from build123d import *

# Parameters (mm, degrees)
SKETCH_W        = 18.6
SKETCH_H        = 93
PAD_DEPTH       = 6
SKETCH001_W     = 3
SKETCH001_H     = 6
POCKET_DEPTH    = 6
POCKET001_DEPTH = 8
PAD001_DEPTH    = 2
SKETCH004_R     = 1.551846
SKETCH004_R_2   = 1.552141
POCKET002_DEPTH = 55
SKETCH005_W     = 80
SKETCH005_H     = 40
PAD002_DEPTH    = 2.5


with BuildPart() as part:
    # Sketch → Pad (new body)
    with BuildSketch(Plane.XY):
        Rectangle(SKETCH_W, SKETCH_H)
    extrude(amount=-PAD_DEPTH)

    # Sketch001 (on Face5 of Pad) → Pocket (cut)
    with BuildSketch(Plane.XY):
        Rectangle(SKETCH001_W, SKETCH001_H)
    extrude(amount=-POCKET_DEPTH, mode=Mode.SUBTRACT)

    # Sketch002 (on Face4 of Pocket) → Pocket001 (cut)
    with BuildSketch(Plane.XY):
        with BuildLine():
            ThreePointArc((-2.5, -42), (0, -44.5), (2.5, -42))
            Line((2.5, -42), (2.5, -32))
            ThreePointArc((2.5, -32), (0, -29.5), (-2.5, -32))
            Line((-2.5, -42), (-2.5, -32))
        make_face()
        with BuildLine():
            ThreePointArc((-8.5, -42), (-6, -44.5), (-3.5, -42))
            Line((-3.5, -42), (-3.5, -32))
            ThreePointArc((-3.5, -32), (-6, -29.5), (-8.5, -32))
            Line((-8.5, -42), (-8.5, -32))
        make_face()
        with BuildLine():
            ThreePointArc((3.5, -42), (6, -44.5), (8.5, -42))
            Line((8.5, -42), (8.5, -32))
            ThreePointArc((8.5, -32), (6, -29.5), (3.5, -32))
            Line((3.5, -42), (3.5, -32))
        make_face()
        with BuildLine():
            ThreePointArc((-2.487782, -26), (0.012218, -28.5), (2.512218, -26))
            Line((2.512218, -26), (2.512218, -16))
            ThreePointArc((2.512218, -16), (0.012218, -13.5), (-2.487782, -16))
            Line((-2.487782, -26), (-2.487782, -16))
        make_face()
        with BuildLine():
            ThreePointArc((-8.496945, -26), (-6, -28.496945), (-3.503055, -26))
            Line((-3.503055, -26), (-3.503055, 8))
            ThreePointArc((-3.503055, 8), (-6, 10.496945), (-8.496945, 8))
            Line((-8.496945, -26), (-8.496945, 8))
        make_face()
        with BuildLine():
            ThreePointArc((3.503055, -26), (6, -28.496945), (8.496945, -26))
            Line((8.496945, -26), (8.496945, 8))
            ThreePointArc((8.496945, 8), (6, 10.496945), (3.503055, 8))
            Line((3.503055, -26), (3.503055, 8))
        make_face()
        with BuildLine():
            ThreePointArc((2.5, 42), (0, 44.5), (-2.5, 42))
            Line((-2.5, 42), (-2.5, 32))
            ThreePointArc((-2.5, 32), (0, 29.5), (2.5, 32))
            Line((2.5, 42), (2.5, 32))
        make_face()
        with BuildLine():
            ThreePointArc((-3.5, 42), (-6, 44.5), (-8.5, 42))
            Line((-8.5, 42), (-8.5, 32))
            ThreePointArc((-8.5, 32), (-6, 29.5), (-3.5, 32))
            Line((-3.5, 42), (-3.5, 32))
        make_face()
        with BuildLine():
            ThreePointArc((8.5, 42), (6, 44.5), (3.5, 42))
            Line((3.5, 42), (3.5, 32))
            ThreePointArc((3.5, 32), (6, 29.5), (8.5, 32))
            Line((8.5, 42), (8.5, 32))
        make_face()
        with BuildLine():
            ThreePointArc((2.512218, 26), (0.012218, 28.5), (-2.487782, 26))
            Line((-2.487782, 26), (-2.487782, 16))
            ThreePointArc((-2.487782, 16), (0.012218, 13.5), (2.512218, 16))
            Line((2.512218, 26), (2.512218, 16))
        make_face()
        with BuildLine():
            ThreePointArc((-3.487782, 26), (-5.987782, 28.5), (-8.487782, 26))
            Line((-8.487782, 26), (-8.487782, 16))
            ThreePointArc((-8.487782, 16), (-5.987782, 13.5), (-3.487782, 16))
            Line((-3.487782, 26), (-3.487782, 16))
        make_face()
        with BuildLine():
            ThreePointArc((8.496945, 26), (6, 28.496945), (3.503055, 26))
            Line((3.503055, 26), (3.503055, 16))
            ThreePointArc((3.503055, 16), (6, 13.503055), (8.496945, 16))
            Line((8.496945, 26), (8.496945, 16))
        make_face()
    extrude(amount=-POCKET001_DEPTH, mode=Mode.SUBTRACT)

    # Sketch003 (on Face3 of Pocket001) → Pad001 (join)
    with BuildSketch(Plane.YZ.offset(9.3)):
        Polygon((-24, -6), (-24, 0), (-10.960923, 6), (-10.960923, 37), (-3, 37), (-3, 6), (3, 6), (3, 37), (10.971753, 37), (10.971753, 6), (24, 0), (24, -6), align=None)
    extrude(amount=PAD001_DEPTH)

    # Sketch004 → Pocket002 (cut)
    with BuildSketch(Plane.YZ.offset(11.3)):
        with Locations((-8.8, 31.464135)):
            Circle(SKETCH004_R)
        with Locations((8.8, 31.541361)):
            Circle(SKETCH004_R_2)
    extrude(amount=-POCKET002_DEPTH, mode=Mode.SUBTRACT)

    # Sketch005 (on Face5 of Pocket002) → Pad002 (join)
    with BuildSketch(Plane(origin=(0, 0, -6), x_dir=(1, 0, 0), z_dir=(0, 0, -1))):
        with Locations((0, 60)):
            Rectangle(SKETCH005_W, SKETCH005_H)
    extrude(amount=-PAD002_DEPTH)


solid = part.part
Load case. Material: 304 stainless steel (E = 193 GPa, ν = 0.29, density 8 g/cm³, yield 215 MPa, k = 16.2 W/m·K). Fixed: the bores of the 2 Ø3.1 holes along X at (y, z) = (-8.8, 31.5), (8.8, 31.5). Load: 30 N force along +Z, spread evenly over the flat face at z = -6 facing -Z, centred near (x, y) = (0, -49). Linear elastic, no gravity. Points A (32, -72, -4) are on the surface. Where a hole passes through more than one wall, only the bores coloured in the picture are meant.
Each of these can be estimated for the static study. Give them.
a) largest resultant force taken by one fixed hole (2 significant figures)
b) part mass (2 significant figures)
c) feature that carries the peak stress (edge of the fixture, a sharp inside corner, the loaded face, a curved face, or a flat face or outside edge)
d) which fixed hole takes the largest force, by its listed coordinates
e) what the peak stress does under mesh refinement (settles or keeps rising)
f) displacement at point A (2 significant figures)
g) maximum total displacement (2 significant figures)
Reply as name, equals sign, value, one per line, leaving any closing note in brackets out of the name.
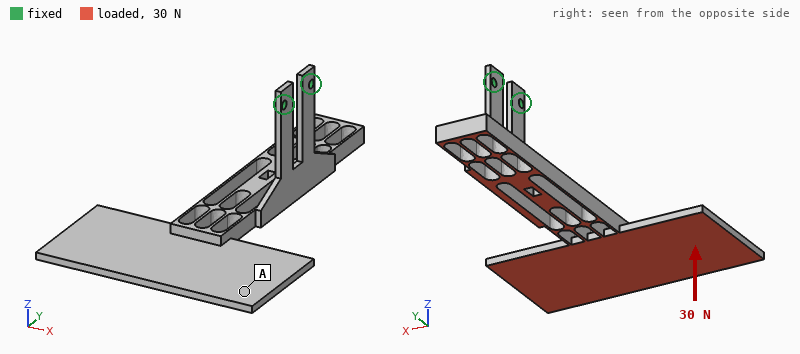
largest resultant force taken by one fixed hole = 110 N
part mass = 110 g
feature that carries the peak stress = a sharp inside corner
which fixed hole takes the largest force, by its listed coordinates = (-8.8, 31.5)
what the peak stress does under mesh refinement = keeps rising
displacement at point A = 0.10 mm
maximum total displacement = 0.47 mm
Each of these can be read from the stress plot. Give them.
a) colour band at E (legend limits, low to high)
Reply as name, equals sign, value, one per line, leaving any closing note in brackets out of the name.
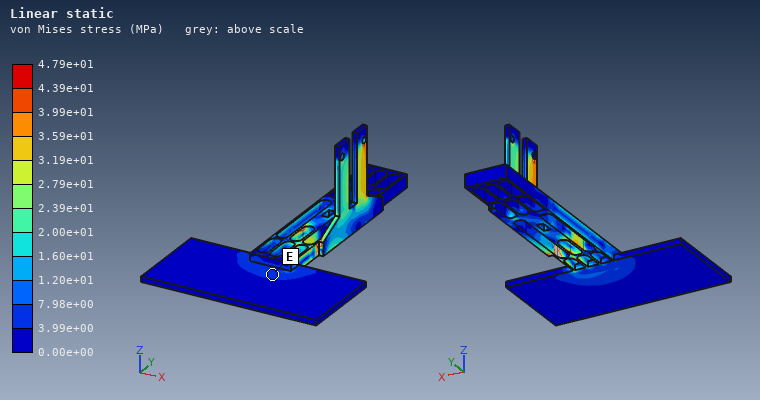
colour band at E = 3.99e+00 to 7.98e+00 MPa
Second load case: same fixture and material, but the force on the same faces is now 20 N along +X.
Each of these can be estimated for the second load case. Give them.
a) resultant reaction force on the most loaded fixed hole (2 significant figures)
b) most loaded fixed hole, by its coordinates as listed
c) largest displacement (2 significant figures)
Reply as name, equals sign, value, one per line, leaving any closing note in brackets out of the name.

resultant reaction force on the most loaded fixed hole = 30 N
most loaded fixed hole, by its coordinates as listed = (-8.8, 31.5)
largest displacement = 0.92 mm
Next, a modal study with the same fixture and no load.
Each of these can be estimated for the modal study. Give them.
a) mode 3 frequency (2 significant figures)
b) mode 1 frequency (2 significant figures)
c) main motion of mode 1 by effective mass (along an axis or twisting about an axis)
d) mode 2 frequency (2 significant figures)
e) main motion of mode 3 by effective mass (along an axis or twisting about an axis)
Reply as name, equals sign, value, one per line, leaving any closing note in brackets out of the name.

mode 3 frequency = 360 Hz
mode 1 frequency = 94 Hz
main motion of mode 1 by effective mass = along X
mode 2 frequency = 150 Hz
main motion of mode 3 by effective mass = along Z
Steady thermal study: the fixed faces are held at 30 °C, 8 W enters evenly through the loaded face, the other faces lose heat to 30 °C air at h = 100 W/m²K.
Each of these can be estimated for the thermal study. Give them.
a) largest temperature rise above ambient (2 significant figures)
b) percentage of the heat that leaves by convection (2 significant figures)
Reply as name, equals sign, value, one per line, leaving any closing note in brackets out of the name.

largest temperature rise above ambient = 17 K
percentage of the heat that leaves by convection = 100 %
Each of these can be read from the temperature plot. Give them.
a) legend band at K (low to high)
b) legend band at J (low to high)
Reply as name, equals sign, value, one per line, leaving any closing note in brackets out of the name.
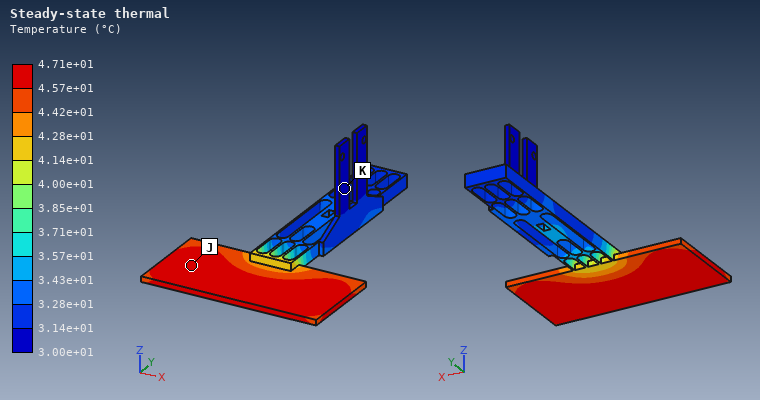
legend band at K = 3.00e+01 to 3.14e+01 °C
legend band at J = 4.57e+01 to 4.71e+01 °C
